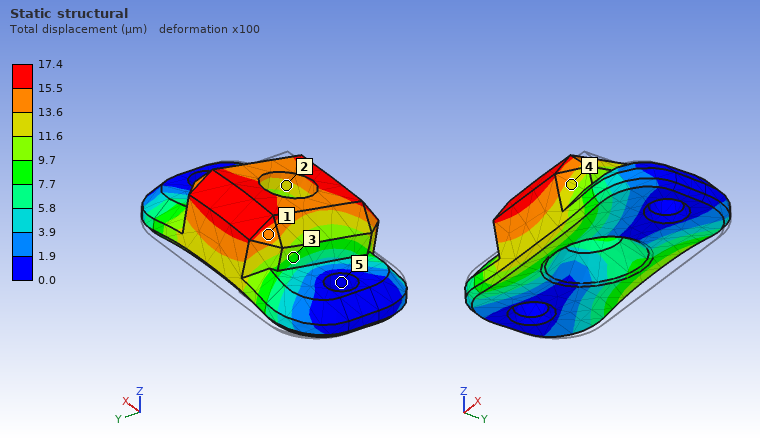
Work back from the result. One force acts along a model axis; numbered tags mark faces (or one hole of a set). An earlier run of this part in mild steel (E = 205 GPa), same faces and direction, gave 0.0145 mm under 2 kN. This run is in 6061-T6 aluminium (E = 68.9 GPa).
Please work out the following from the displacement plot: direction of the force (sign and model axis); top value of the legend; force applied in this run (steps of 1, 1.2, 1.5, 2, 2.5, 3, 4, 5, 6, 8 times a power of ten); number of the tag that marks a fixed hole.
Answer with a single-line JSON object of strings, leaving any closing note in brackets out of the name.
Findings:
{"direction of the force": "-Y", "top value of the legend": "17.4 µm", "force applied in this run": "800 N", "number of the tag that marks a fixed hole": "5"}
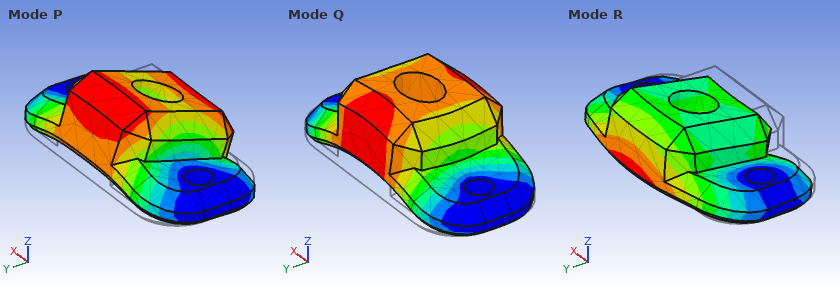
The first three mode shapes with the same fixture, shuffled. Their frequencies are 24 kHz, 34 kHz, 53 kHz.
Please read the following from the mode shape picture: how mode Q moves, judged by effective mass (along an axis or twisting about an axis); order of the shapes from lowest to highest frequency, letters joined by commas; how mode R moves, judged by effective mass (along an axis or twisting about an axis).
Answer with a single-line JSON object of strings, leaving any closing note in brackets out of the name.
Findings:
{"how mode Q moves, judged by effective mass": "along Z", "order of the shapes from lowest to highest frequency, letters joined by commas": "P, Q, R", "how mode R moves, judged by effective mass": "along Y"}
